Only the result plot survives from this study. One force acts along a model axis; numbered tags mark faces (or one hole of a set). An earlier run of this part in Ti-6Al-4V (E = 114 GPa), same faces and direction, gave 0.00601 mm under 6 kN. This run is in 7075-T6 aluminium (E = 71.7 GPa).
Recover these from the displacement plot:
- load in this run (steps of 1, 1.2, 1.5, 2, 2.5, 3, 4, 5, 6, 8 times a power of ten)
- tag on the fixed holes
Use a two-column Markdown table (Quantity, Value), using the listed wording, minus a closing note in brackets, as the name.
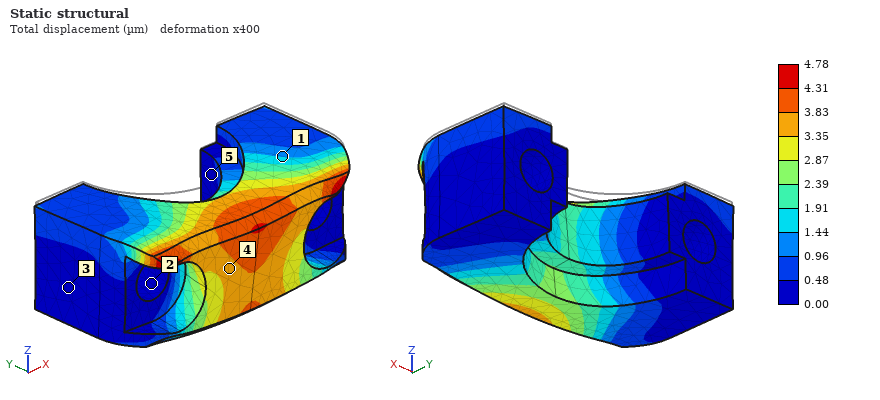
| Quantity | Value |
|---|---|
| load in this run | 3 kN |
| tag on the fixed holes | 2 |
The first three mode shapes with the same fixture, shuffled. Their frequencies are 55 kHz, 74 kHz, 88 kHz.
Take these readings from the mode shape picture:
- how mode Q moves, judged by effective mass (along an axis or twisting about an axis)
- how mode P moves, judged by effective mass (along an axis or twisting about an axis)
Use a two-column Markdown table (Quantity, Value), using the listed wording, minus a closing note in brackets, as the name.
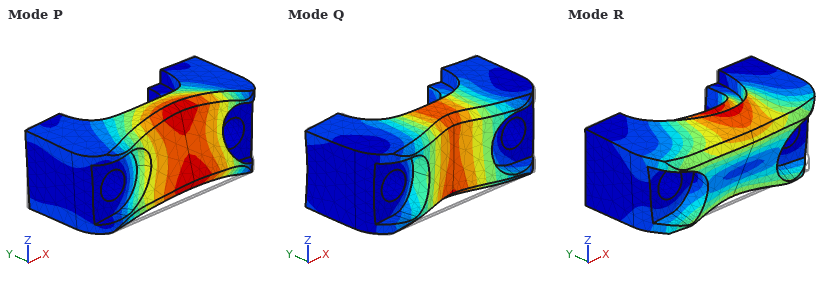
| Quantity | Value |
|---|---|
| how mode Q moves, judged by effective mass | along Y |
| how mode P moves, judged by effective mass | along Z |
